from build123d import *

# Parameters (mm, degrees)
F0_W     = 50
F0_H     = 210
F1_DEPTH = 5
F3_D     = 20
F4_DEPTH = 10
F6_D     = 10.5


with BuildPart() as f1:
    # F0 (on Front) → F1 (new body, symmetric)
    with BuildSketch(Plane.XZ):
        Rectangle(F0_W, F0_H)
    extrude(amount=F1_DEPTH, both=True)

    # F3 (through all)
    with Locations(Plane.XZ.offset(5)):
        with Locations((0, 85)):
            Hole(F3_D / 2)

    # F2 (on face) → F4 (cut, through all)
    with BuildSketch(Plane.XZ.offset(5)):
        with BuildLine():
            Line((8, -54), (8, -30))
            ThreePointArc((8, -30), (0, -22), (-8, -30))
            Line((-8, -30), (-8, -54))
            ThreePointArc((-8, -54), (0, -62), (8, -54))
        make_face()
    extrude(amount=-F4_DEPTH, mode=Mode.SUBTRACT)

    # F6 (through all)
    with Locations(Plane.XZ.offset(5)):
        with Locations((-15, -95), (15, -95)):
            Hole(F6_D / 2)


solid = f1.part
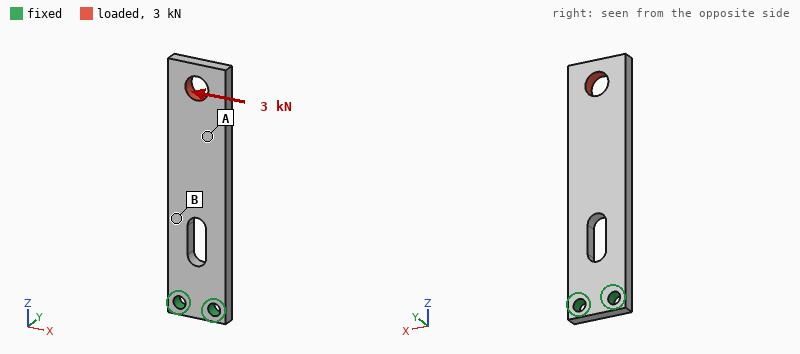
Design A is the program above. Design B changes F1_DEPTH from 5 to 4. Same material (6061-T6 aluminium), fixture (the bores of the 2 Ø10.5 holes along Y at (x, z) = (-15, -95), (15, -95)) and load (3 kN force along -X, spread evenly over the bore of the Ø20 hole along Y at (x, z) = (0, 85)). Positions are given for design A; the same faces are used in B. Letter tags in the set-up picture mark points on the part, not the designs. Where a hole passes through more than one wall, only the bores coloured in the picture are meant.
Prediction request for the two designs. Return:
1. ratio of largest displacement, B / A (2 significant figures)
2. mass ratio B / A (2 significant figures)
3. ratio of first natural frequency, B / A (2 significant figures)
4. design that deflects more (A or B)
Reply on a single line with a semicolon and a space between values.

1.3; 0.80; 0.80; B
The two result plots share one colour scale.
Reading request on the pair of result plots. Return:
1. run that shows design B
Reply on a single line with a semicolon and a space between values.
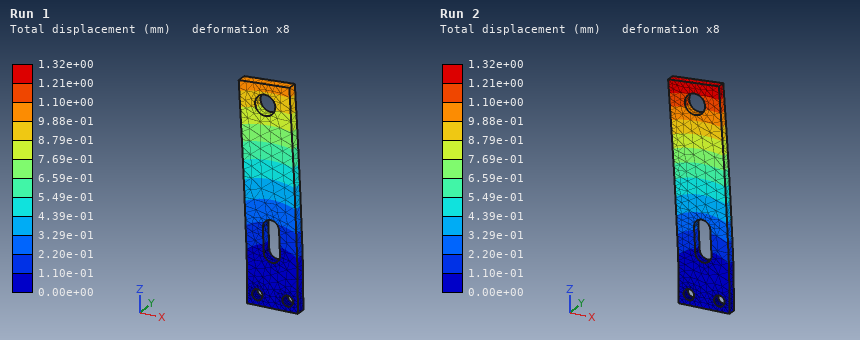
Run 2
